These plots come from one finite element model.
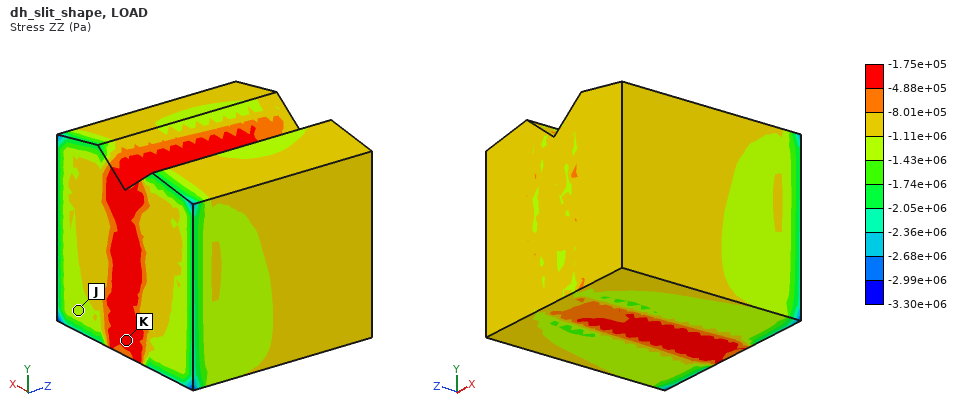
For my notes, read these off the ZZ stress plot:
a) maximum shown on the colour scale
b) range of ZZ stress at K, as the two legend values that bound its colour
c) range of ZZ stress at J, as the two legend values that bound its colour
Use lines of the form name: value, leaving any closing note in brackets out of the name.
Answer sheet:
maximum shown on the colour scale: -1.75e+05 Pa
range of ZZ stress at K, as the two legend values that bound its colour: -4.88e+05 to -1.75e+05 Pa
range of ZZ stress at J, as the two legend values that bound its colour: -1.43e+06 to -1.11e+06 Pa
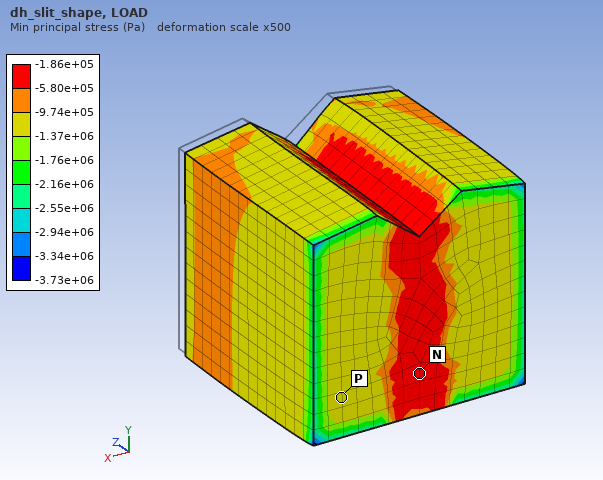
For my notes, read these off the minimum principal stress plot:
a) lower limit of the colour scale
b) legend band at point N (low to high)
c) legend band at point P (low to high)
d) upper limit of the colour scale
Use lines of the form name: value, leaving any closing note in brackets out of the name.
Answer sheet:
lower limit of the colour scale: -3.73e+06 Pa
legend band at point N: -5.80e+05 to -1.86e+05 Pa
legend band at point P: -1.37e+06 to -9.74e+05 Pa
upper limit of the colour scale: -1.86e+05 Pa
